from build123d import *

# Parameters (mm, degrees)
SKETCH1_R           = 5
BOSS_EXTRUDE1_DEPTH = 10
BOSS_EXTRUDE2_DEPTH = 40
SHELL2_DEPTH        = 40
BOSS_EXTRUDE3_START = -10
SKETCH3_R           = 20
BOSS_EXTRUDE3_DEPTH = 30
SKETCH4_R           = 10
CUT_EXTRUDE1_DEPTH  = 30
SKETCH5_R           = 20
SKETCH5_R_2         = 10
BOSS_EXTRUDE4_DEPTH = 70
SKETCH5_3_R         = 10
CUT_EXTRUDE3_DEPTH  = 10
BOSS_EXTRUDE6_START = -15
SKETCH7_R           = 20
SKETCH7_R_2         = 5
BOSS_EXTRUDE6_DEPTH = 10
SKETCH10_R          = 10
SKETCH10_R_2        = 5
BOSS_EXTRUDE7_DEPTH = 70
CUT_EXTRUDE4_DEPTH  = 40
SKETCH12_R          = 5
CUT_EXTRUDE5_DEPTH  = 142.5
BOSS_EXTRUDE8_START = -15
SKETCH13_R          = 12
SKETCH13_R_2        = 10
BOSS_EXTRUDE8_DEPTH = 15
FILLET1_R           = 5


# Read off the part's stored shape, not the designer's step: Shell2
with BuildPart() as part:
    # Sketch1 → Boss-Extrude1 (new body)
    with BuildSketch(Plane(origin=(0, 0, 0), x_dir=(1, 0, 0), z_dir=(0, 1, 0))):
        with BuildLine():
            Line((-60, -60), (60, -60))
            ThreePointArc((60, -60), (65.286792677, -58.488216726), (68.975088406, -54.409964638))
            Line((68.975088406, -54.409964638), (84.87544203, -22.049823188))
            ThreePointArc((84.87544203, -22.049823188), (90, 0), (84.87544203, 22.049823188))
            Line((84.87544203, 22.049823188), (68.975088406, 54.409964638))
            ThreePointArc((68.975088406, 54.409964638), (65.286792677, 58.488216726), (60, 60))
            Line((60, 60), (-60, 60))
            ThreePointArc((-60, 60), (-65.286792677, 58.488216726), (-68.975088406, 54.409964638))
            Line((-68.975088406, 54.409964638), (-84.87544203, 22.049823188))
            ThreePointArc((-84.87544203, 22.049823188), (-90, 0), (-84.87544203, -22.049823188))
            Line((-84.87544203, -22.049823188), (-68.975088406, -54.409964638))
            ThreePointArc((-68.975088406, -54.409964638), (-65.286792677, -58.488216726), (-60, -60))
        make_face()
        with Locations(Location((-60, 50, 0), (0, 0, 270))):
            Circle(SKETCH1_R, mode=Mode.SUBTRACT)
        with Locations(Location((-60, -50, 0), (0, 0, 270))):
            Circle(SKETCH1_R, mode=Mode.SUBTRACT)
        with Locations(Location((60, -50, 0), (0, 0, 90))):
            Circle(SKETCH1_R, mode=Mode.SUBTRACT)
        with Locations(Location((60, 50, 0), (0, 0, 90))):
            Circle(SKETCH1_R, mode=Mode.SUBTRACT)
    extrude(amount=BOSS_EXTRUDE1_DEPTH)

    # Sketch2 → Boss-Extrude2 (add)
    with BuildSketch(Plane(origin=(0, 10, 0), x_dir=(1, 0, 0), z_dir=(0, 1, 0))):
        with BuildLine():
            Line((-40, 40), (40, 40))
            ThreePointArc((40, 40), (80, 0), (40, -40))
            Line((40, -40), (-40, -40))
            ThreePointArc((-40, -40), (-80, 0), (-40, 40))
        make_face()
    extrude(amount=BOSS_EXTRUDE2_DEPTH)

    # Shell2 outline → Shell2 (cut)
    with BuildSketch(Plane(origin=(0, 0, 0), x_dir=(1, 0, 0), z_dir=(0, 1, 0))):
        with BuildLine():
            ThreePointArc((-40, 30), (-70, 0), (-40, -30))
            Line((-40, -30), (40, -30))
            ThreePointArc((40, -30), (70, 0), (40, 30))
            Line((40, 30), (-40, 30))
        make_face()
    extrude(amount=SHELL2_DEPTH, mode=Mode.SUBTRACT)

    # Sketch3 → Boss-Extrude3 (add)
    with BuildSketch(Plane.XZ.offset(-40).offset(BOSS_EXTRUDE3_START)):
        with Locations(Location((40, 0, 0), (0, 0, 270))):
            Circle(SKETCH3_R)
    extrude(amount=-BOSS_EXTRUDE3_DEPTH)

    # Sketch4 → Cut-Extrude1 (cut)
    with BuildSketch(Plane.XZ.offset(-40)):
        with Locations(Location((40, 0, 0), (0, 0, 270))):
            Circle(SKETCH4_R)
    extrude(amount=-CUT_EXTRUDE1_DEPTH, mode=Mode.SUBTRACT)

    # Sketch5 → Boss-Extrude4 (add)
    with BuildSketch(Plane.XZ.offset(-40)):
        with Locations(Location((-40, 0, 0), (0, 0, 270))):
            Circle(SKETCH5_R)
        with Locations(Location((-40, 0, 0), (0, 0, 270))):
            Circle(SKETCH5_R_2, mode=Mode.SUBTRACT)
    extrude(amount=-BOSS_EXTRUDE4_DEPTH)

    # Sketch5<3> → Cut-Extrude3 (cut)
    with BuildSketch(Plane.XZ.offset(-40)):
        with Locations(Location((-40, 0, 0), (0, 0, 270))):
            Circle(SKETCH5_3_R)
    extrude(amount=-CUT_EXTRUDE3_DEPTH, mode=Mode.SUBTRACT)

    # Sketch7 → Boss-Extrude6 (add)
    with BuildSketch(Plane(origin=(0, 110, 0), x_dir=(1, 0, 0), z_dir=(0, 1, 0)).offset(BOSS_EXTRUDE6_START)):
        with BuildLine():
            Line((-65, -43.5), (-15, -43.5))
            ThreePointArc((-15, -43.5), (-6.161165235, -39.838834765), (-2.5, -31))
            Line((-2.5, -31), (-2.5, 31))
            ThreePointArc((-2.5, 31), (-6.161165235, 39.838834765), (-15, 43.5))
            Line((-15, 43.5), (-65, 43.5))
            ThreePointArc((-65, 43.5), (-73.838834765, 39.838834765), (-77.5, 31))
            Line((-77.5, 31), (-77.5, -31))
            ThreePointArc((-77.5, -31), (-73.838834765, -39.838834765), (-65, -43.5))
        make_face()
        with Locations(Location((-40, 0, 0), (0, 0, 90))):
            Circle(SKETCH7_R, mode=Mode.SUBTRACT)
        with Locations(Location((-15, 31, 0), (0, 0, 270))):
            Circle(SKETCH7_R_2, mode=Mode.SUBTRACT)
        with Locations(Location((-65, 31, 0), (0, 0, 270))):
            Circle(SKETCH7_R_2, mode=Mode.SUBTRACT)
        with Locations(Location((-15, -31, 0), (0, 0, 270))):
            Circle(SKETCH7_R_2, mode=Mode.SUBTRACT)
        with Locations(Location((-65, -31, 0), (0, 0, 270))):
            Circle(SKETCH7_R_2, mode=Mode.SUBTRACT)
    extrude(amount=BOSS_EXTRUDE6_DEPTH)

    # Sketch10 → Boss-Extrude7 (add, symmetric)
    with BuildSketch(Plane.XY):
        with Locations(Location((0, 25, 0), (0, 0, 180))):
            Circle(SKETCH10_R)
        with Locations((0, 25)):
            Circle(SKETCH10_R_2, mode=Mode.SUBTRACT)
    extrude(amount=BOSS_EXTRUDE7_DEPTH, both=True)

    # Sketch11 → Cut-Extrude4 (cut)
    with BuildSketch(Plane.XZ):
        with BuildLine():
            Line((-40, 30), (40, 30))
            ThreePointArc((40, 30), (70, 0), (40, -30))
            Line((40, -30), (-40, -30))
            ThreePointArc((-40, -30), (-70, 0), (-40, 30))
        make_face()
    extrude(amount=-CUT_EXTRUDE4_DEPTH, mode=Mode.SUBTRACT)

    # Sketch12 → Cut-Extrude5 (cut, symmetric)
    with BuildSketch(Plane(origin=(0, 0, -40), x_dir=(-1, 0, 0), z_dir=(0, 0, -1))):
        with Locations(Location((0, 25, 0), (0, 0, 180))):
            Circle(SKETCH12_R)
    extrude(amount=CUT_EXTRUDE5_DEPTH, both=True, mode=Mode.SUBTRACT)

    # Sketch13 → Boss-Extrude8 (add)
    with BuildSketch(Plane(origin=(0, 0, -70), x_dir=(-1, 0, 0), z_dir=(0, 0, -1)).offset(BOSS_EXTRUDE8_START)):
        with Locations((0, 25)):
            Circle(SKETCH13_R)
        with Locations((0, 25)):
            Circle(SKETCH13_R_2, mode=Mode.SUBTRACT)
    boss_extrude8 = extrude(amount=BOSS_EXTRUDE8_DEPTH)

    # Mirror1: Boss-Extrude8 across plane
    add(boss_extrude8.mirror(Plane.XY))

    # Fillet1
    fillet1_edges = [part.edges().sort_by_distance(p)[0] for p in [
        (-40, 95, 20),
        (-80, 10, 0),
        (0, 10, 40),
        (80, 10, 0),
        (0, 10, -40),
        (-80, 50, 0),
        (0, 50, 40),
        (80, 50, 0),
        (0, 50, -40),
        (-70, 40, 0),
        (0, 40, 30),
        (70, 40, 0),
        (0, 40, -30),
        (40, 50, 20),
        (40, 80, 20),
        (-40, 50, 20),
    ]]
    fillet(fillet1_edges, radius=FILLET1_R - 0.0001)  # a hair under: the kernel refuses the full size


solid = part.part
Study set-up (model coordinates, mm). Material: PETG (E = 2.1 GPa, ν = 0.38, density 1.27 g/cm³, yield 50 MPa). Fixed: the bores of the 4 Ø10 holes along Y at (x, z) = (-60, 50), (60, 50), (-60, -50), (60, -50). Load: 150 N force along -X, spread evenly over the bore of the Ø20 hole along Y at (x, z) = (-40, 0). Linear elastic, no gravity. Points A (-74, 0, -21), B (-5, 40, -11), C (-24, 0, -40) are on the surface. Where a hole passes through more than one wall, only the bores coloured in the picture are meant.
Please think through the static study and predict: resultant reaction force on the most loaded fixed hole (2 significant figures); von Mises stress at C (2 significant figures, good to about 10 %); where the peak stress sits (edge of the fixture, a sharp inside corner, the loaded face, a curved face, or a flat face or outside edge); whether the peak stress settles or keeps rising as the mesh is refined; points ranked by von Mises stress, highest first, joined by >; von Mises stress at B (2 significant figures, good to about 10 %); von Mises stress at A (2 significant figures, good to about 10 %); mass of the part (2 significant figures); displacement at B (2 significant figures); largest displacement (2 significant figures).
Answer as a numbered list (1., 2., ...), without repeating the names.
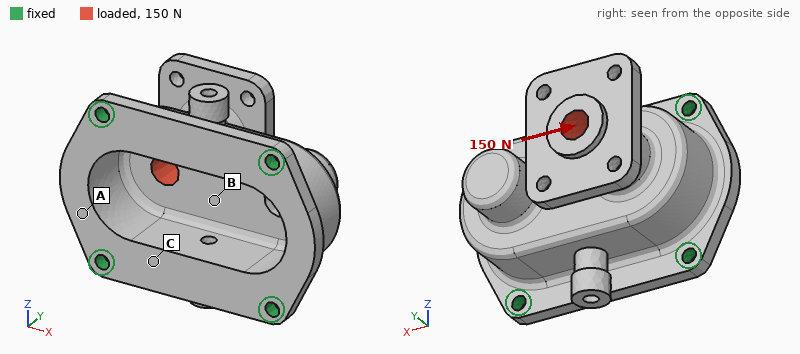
1. 71 N
2. 0.10 MPa
3. edge of the fixture
4. keeps rising
5. B > A > C
6. 0.32 MPa
7. 0.22 MPa
8. 620 g
9. 18 µm
10. 88 µm
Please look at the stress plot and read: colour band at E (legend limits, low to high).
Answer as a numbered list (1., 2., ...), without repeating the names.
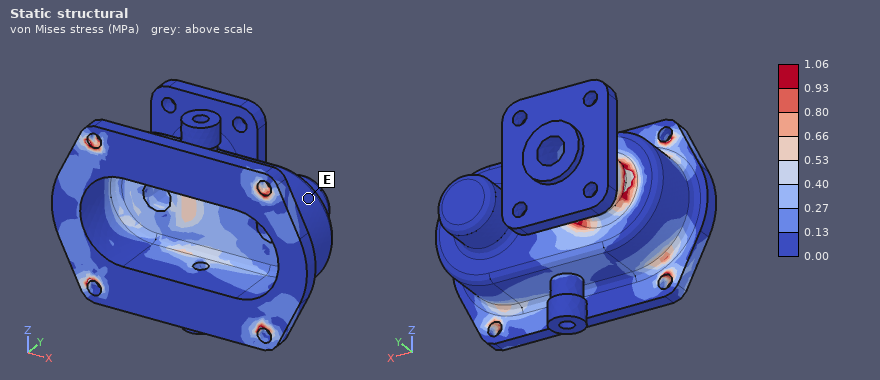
1. 0.00 to 0.13 MPa
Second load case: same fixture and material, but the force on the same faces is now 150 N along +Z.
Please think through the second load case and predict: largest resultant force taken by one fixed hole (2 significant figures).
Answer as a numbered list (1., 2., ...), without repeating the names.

1. 94 N
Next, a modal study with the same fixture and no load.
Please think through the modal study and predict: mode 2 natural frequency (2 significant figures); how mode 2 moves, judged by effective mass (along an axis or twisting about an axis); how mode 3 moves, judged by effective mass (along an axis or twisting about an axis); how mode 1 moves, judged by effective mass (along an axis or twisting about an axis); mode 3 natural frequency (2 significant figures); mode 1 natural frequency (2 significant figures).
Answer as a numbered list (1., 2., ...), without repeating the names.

1. 520 Hz
2. along Z
3. along Y
4. along X
5. 880 Hz
6. 500 Hz
